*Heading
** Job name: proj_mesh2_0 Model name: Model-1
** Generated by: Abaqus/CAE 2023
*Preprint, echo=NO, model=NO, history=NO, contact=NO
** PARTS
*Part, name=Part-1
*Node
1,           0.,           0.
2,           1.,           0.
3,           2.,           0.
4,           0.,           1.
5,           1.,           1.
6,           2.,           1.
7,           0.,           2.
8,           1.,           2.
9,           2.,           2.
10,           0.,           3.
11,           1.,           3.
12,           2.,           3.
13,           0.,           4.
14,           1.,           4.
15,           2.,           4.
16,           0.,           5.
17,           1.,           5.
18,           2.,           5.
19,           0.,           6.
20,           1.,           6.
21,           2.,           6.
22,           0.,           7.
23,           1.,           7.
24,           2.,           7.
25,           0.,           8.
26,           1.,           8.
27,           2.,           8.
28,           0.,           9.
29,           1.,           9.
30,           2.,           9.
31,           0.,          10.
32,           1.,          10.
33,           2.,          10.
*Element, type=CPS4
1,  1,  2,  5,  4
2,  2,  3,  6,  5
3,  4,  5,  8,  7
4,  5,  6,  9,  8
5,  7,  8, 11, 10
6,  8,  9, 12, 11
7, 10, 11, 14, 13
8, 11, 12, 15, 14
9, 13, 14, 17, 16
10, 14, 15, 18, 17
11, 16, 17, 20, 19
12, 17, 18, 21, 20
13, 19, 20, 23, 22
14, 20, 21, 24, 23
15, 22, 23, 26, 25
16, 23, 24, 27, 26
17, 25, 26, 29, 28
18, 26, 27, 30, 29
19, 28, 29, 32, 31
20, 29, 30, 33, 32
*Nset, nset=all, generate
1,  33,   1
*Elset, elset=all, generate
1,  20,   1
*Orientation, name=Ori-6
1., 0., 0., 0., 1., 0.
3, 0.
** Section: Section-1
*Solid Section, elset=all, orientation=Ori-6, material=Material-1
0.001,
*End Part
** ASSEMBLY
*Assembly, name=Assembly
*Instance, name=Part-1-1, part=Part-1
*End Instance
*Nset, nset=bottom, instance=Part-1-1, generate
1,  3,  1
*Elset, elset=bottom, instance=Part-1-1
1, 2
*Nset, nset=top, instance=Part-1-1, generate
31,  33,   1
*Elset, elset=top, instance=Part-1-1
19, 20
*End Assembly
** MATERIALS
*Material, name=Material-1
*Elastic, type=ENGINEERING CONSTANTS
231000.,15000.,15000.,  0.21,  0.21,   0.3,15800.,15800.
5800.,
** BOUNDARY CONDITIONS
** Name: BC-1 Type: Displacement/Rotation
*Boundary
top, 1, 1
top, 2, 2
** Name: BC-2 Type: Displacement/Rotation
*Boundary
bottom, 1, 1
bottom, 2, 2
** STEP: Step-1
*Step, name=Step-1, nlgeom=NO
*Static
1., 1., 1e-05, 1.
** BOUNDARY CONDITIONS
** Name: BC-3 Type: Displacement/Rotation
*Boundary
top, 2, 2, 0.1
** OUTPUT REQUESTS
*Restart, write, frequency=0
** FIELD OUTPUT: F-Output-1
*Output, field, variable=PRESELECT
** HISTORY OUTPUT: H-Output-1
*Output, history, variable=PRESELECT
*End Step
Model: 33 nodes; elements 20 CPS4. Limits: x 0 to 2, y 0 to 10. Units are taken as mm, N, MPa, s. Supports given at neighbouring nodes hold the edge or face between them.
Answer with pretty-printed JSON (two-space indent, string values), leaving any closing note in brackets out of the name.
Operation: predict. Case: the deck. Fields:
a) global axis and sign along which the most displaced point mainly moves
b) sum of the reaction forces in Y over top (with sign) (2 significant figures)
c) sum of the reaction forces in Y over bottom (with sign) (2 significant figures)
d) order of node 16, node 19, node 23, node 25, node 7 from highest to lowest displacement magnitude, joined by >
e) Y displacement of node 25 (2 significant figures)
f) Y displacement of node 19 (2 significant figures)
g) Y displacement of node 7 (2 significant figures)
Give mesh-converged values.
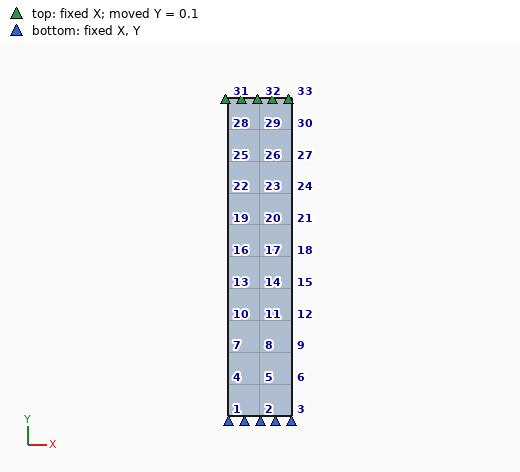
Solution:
{
  "global axis and sign along which the most displaced point mainly moves": "+Y",
  "sum of the reaction forces in Y over top (with sign)": "0.30 N",
  "sum of the reaction forces in Y over bottom (with sign)": "-0.30 N",
  "order of node 16, node 19, node 23, node 25, node 7 from highest to lowest displacement magnitude, joined by >": "node 25 > node 23 > node 19 > node 16 > node 7",
  "Y displacement of node 25": "0.080 mm",
  "Y displacement of node 19": "0.060 mm",
  "Y displacement of node 7": "0.020 mm"
}
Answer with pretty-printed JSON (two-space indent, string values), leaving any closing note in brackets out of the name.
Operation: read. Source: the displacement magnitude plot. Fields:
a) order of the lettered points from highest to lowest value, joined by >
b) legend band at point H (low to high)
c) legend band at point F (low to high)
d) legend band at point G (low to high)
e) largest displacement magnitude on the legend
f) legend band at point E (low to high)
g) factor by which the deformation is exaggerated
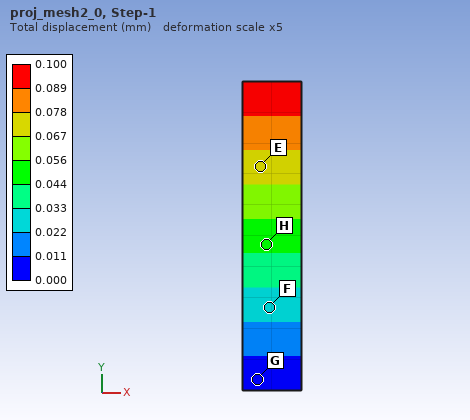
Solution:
{
  "order of the lettered points from highest to lowest value, joined by >": "E > H > F > G",
  "legend band at point H": "0.044 to 0.056 mm",
  "legend band at point F": "0.022 to 0.033 mm",
  "legend band at point G": "0.000 to 0.011 mm",
  "largest displacement magnitude on the legend": "0.100 mm",
  "legend band at point E": "0.067 to 0.078 mm",
  "factor by which the deformation is exaggerated": "5"
}
